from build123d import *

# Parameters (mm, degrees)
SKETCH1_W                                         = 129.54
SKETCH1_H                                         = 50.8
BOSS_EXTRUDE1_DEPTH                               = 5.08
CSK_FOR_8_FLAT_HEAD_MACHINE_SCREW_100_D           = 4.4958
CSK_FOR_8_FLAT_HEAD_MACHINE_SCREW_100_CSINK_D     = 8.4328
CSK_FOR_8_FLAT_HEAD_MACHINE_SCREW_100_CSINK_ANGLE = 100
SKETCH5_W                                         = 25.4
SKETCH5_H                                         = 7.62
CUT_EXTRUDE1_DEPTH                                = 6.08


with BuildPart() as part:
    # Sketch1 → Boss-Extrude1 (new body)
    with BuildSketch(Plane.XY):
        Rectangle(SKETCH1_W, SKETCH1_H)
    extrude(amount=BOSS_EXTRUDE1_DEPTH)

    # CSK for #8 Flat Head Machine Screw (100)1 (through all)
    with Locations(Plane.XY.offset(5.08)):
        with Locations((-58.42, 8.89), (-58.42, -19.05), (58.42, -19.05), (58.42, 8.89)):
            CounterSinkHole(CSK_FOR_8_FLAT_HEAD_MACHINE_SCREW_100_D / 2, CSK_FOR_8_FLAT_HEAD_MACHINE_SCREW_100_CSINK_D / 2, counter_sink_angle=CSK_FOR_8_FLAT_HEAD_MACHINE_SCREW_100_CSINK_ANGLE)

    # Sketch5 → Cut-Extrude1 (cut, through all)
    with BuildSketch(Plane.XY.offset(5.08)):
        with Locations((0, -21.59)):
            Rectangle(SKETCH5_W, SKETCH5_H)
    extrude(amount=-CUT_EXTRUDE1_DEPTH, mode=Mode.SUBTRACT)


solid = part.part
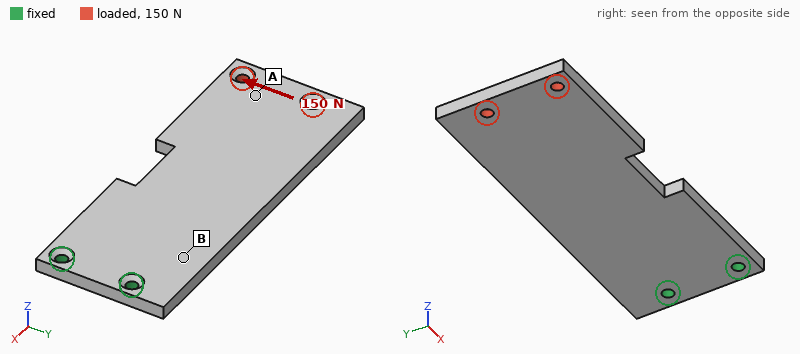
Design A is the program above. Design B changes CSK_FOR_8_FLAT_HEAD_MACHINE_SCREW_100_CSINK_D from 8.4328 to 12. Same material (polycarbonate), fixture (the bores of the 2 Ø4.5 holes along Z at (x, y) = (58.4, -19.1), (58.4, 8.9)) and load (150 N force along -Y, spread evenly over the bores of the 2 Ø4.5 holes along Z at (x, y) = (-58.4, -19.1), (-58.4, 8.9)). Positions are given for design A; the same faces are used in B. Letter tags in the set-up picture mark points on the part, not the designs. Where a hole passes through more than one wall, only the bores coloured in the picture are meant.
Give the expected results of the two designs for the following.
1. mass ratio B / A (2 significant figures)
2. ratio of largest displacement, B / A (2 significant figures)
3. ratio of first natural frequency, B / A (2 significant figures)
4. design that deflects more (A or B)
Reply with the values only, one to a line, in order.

0.99
1.3
0.89
B
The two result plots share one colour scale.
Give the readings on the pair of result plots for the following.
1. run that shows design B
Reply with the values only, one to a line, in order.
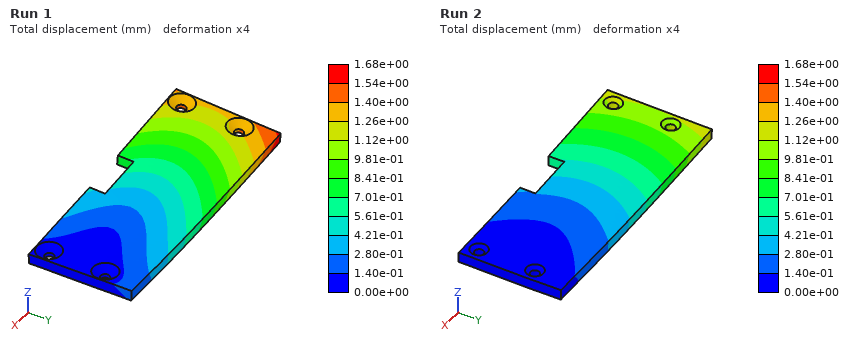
Run 1
